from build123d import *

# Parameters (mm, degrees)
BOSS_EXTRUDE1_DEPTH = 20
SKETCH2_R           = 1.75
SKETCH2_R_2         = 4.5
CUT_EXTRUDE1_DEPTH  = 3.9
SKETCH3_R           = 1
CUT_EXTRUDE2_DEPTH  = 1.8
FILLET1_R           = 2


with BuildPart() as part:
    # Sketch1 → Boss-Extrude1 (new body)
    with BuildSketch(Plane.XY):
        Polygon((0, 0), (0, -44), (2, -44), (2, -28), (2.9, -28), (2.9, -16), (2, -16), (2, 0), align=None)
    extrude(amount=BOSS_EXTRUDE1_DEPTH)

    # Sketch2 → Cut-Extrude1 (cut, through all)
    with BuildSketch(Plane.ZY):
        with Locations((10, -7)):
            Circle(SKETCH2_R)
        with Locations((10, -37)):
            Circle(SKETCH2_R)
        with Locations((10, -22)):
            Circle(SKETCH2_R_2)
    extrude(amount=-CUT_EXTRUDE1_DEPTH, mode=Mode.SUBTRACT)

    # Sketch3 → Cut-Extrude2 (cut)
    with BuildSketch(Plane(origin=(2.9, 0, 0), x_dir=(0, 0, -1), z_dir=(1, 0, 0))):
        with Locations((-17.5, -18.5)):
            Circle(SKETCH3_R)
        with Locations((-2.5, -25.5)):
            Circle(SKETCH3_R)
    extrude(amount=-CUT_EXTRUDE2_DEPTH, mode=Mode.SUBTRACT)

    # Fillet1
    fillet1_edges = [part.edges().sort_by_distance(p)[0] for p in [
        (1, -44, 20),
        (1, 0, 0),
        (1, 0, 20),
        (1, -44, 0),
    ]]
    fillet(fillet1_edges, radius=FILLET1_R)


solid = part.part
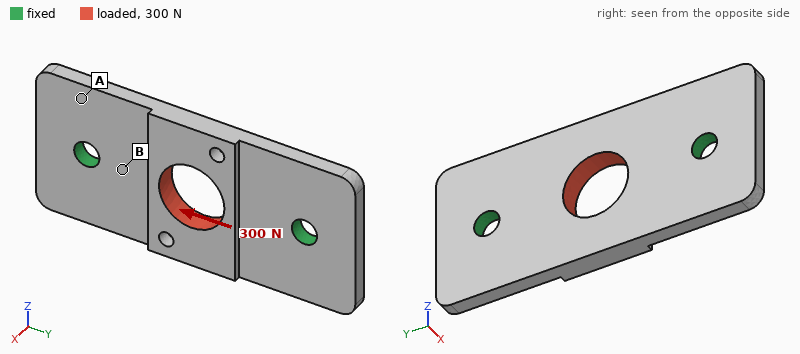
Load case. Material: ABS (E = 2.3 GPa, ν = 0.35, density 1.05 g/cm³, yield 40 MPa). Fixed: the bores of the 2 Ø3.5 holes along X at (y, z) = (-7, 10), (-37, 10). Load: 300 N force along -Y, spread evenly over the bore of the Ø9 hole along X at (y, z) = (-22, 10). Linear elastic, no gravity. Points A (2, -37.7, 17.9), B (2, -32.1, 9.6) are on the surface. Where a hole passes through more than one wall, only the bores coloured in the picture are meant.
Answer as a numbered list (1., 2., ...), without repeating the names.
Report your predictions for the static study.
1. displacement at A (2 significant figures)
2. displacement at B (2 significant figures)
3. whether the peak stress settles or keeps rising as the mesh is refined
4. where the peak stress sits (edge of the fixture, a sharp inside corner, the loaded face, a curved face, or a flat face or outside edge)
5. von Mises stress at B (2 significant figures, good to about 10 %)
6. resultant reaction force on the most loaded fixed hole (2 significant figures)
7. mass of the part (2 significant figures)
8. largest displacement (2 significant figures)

1. 17 µm
2. 12 µm
3. keeps rising
4. edge of the fixture
5. 9.1 MPa
6. 150 N
7. 1.8 g
8. 38 µm
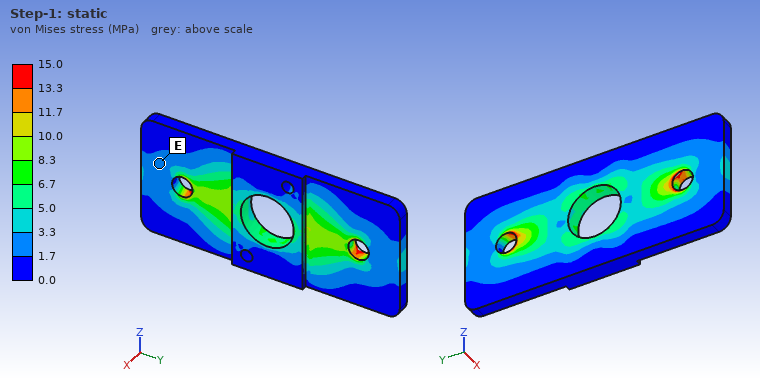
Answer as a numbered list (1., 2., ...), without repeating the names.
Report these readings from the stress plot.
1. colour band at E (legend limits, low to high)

1. 1.7 to 3.3 MPa
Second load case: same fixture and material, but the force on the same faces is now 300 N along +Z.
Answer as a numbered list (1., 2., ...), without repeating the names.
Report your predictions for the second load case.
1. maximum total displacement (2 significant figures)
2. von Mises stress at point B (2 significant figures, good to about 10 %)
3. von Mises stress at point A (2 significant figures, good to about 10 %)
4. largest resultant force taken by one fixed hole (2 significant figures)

1. 0.19 mm
2. 13 MPa
3. 2.4 MPa
4. 150 N
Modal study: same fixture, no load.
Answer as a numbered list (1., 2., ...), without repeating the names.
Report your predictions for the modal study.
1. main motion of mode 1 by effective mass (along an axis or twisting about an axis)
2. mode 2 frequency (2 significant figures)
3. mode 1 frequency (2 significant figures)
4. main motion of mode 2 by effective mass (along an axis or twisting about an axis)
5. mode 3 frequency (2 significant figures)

1. twisting about Y
2. 3300 Hz
3. 2900 Hz
4. along X
5. 5500 Hz
